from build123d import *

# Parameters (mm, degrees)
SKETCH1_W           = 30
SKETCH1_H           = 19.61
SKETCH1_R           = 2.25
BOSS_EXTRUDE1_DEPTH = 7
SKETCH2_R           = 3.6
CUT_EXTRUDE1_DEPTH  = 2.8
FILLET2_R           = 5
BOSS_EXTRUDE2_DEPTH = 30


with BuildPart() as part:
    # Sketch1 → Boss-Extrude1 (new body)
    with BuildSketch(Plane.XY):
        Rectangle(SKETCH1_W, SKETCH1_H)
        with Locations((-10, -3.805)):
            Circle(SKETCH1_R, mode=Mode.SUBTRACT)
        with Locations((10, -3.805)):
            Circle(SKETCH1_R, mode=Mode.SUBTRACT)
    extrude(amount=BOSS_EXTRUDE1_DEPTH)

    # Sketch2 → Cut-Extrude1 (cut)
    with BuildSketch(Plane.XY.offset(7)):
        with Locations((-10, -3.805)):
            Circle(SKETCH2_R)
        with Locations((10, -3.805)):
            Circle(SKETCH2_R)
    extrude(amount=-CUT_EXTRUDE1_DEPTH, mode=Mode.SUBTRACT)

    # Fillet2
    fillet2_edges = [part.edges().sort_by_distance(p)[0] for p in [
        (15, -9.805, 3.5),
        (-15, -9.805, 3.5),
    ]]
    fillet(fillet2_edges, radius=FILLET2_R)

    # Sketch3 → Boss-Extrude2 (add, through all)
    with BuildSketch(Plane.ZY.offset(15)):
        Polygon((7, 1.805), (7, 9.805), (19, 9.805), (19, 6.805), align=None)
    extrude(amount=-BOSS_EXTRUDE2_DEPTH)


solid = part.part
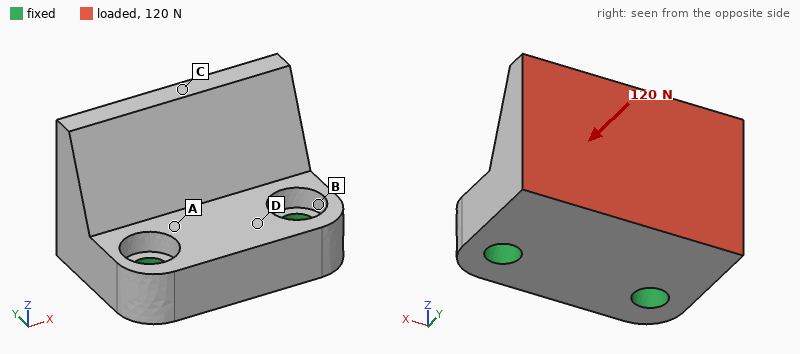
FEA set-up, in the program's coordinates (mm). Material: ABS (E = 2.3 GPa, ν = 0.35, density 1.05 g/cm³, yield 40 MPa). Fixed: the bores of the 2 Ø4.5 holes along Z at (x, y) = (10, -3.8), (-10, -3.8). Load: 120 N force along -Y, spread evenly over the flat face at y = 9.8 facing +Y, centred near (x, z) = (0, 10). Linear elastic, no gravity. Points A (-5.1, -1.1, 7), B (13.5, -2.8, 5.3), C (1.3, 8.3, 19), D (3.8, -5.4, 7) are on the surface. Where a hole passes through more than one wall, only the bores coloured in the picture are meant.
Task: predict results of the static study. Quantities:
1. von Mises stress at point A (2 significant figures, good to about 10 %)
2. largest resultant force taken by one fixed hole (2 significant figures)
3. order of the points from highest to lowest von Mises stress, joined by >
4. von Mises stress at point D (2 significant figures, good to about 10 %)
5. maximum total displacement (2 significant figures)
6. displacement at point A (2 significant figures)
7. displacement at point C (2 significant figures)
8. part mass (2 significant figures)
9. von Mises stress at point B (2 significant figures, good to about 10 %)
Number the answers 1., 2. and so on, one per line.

1. 3.5 MPa
2. 61 N
3. B > A > D > C
4. 1.7 MPa
5. 0.14 mm
6. 0.023 mm
7. 0.13 mm
8. 5.9 g
9. 6.1 MPa
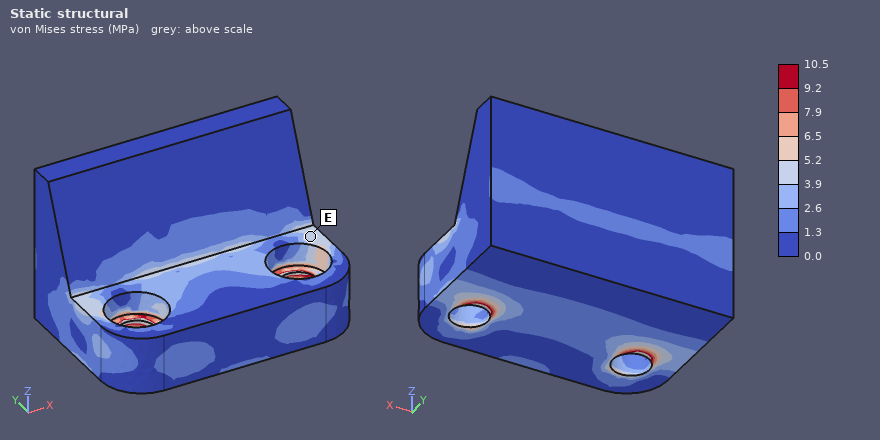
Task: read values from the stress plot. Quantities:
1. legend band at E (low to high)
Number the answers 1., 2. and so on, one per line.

1. 3.9 to 5.2 MPa
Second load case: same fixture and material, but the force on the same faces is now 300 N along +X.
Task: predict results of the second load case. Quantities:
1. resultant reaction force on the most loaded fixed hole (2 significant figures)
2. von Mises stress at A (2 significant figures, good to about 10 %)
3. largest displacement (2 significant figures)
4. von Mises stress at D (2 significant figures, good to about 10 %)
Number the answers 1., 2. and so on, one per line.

1. 250 N
2. 2.9 MPa
3. 74 µm
4. 1.4 MPa
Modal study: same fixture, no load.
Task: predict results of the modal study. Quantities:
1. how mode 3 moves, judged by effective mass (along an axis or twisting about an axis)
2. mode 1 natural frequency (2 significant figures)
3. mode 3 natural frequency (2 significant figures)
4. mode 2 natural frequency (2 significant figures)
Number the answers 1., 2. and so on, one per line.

1. along X
2. 2700 Hz
3. 7900 Hz
4. 5300 Hz
